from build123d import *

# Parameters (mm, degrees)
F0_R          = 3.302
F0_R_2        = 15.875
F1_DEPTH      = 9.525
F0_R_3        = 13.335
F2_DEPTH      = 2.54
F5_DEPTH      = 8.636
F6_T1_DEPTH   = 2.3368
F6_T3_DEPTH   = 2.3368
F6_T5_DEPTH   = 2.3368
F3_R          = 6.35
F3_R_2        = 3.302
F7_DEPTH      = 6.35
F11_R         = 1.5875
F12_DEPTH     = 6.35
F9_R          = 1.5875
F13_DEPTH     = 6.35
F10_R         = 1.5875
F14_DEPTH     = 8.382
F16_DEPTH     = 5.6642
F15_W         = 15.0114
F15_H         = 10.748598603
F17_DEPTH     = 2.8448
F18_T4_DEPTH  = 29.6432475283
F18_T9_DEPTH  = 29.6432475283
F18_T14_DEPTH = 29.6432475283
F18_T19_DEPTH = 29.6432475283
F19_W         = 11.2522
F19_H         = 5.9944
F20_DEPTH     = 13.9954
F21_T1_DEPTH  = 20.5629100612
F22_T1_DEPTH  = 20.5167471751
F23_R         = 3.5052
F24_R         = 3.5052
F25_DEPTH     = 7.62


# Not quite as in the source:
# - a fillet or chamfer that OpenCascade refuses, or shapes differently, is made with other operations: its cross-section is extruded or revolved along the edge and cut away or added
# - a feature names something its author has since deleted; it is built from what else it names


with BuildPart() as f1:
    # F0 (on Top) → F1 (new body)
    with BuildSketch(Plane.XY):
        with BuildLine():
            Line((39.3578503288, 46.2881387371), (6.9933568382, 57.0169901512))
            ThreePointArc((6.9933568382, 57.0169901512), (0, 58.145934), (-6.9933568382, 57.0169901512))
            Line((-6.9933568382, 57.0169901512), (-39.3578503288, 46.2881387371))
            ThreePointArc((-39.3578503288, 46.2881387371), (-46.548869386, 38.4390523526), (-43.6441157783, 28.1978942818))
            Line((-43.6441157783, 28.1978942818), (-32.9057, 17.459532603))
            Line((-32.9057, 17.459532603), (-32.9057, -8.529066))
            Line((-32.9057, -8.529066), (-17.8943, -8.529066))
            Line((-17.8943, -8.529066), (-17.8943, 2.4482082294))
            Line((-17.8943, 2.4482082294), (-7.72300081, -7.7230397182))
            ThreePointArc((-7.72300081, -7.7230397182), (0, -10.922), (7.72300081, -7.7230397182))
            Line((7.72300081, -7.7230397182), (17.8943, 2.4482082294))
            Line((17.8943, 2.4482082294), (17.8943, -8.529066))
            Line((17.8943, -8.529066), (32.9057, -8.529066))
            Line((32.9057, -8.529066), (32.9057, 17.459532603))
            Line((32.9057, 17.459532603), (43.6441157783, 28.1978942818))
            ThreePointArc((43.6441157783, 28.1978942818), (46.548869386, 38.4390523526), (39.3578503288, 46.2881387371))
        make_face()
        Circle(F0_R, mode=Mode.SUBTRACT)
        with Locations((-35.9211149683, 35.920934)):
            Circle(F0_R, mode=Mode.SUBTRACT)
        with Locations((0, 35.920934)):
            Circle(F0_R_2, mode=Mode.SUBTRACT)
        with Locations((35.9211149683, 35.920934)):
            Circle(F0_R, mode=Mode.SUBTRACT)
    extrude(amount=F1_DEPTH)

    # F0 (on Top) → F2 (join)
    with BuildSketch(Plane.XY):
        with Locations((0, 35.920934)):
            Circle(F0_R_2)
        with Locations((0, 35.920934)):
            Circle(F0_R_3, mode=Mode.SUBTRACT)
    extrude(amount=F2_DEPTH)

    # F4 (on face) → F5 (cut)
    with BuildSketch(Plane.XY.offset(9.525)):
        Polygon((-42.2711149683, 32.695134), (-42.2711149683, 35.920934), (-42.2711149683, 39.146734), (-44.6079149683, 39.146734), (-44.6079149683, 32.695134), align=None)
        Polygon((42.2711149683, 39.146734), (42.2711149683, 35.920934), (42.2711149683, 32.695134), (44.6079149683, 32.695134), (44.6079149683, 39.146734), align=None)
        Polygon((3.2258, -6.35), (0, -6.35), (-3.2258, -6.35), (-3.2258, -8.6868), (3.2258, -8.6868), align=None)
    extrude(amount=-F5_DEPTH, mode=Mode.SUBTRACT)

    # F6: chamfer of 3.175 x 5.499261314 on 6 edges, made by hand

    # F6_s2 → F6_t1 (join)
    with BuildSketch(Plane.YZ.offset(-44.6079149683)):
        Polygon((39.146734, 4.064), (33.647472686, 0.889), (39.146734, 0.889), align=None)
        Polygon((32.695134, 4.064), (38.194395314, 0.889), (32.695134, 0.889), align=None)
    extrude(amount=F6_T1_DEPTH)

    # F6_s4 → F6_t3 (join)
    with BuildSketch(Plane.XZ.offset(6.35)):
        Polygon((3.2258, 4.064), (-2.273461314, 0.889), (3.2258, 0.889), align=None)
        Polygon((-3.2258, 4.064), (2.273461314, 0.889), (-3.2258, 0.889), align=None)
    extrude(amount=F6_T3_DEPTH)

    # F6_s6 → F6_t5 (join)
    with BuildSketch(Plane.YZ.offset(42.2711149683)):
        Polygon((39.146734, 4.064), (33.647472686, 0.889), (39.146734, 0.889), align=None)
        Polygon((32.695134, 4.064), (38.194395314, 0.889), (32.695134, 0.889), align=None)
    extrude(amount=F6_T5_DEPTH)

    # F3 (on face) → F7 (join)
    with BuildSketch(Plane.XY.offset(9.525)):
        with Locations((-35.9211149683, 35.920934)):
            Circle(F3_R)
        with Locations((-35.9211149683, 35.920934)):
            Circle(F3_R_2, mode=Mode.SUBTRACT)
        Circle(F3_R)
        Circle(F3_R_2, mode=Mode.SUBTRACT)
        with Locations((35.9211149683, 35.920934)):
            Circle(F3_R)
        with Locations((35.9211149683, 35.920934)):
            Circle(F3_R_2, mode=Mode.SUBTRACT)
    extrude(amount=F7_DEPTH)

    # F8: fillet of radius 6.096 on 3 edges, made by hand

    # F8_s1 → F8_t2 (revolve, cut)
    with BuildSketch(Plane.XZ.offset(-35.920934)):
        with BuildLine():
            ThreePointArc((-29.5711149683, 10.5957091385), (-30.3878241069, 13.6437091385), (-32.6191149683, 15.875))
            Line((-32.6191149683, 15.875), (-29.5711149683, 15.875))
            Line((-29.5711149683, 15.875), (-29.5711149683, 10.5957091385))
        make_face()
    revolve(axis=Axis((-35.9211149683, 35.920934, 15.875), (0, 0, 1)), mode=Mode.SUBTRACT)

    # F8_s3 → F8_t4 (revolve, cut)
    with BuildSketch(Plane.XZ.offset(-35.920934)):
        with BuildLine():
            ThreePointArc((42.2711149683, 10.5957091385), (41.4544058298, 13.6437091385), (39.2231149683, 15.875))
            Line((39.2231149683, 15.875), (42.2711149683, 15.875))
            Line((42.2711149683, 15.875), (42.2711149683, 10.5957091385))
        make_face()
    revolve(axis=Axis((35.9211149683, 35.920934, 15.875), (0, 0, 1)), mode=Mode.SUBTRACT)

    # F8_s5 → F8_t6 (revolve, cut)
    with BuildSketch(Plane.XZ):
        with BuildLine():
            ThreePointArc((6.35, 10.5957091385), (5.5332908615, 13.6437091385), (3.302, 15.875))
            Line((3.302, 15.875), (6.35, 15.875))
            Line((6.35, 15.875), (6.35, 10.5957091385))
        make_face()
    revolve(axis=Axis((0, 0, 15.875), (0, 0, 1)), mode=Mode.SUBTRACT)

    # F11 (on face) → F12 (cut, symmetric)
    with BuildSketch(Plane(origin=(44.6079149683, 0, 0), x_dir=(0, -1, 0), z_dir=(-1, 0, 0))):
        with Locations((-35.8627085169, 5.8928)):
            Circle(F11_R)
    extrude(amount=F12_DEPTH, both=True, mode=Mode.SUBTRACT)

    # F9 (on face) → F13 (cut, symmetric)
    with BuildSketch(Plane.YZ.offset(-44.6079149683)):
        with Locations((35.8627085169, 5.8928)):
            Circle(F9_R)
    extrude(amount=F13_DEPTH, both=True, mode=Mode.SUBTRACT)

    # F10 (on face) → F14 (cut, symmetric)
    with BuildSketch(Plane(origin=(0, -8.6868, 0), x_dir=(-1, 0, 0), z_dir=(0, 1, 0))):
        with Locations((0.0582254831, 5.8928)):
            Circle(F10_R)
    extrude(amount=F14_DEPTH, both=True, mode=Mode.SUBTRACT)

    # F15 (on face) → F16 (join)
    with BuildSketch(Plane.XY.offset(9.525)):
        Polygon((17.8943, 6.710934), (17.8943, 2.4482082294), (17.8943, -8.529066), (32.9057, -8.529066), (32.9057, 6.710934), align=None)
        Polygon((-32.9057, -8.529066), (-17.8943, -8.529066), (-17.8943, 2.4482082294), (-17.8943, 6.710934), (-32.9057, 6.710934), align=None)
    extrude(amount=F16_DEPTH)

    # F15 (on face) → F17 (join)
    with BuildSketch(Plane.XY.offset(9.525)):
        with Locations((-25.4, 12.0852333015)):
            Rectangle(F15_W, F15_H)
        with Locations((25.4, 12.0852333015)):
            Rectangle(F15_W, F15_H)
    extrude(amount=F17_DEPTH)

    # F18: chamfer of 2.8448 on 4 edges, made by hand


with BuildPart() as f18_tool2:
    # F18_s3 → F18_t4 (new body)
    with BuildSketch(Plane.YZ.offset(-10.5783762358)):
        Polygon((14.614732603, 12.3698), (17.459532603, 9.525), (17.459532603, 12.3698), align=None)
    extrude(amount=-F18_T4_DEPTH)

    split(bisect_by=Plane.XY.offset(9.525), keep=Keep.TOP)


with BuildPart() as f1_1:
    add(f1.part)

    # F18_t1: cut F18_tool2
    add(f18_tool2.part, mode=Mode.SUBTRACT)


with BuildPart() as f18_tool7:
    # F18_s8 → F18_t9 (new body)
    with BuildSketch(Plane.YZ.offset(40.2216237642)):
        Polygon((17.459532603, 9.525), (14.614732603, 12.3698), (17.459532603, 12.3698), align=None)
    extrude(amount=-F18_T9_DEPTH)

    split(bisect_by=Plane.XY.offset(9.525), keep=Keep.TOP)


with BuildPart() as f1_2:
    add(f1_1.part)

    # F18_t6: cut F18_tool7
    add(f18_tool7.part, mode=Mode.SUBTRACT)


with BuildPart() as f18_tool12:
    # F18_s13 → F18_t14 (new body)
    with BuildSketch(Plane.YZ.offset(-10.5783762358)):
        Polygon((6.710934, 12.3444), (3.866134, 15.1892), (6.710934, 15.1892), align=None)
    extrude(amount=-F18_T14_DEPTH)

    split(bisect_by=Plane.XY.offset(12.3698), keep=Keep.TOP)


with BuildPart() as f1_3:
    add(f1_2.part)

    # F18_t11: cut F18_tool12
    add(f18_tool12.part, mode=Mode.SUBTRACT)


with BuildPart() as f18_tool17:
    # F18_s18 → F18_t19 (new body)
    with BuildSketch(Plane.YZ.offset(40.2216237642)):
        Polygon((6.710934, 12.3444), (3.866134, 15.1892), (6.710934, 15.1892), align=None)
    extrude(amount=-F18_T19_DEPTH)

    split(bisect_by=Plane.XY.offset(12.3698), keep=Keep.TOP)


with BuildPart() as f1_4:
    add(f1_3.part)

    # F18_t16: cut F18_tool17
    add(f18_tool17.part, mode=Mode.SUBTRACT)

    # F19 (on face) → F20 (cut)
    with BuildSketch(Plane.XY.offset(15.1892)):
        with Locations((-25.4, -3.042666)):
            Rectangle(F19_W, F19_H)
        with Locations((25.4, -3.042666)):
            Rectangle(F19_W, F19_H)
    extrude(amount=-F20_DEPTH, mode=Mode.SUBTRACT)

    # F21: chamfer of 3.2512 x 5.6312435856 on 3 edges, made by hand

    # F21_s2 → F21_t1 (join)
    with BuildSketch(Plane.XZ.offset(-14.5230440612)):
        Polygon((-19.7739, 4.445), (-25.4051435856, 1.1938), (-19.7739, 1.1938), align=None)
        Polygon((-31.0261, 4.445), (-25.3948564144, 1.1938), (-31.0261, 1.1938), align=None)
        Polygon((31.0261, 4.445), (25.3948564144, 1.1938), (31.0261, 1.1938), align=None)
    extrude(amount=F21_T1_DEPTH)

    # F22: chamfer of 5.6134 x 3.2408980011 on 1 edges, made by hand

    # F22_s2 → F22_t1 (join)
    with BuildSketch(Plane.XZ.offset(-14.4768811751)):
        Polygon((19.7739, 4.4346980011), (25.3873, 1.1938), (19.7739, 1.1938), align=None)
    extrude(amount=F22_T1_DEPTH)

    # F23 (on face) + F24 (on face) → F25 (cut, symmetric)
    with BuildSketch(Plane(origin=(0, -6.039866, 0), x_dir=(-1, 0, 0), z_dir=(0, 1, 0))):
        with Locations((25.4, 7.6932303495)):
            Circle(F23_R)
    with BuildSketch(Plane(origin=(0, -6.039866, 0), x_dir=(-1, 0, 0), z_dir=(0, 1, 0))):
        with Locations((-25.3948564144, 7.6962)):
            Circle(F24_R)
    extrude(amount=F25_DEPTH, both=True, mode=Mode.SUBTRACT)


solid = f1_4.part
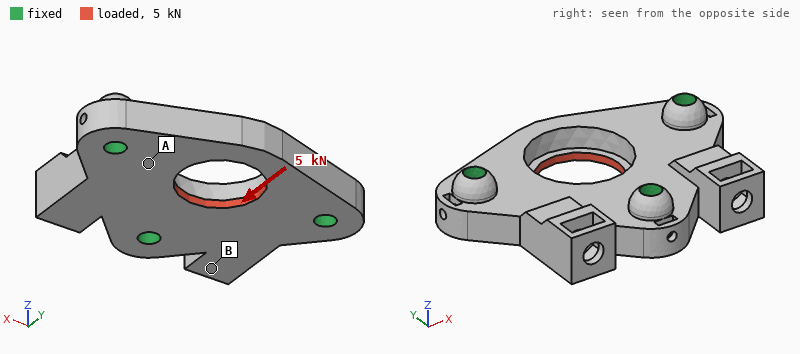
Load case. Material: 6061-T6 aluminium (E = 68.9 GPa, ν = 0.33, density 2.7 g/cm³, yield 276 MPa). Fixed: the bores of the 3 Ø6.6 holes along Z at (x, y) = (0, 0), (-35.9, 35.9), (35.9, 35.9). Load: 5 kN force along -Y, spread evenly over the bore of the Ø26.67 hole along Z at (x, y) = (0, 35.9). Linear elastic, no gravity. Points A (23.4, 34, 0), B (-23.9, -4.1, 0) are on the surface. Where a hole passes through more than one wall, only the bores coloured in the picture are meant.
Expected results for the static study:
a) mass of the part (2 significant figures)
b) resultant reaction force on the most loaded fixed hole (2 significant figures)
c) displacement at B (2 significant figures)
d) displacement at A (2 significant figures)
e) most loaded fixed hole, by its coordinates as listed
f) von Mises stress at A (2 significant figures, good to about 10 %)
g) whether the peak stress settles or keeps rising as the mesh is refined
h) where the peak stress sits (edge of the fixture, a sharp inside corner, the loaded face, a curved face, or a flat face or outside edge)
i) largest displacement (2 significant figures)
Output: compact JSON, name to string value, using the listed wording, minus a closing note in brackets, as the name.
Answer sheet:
{"mass of the part": "100 g", "resultant reaction force on the most loaded fixed hole": "2.2 kN", "displacement at B": "4.6 µm", "displacement at A": "4.9 µm", "most loaded fixed hole, by its coordinates as listed": "(0, 0)", "von Mises stress at A": "12 MPa", "whether the peak stress settles or keeps rising as the mesh is refined": "keeps rising", "where the peak stress sits": "a sharp inside corner", "largest displacement": "30 µm"}
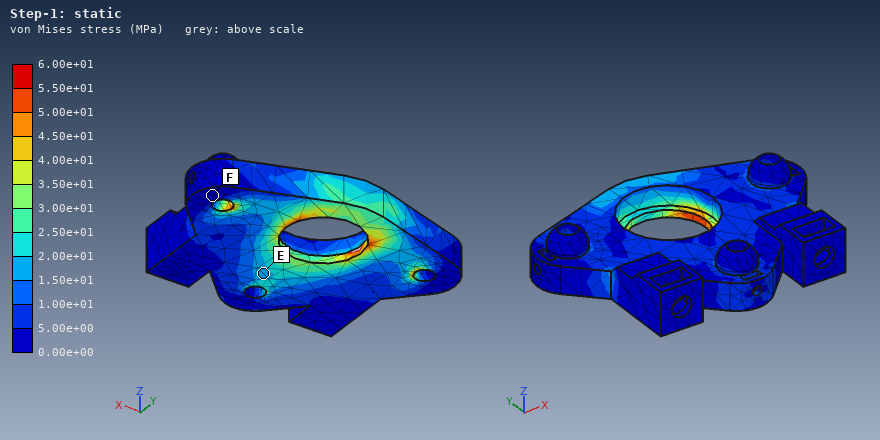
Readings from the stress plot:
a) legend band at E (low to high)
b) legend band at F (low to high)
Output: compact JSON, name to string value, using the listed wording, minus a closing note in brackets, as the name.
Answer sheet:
{"legend band at E": "1.50e+01 to 2.00e+01 MPa", "legend band at F": "0.00e+00 to 5.00e+00 MPa"}
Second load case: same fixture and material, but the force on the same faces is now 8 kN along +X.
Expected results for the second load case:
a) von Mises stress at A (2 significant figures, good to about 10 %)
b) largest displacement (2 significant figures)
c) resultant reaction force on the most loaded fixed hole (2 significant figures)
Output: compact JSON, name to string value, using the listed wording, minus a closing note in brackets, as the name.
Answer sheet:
{"von Mises stress at A": "29 MPa", "largest displacement": "16 µm", "resultant reaction force on the most loaded fixed hole": "3.4 kN"}
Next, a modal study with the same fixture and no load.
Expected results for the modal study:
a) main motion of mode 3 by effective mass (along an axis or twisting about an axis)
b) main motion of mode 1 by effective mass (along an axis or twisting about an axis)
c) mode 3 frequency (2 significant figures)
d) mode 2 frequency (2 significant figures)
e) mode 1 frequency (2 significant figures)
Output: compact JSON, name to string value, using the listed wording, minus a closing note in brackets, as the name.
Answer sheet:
{"main motion of mode 3 by effective mass": "along Z", "main motion of mode 1 by effective mass": "twisting about X", "mode 3 frequency": "9900 Hz", "mode 2 frequency": "9000 Hz", "mode 1 frequency": "8600 Hz"}
